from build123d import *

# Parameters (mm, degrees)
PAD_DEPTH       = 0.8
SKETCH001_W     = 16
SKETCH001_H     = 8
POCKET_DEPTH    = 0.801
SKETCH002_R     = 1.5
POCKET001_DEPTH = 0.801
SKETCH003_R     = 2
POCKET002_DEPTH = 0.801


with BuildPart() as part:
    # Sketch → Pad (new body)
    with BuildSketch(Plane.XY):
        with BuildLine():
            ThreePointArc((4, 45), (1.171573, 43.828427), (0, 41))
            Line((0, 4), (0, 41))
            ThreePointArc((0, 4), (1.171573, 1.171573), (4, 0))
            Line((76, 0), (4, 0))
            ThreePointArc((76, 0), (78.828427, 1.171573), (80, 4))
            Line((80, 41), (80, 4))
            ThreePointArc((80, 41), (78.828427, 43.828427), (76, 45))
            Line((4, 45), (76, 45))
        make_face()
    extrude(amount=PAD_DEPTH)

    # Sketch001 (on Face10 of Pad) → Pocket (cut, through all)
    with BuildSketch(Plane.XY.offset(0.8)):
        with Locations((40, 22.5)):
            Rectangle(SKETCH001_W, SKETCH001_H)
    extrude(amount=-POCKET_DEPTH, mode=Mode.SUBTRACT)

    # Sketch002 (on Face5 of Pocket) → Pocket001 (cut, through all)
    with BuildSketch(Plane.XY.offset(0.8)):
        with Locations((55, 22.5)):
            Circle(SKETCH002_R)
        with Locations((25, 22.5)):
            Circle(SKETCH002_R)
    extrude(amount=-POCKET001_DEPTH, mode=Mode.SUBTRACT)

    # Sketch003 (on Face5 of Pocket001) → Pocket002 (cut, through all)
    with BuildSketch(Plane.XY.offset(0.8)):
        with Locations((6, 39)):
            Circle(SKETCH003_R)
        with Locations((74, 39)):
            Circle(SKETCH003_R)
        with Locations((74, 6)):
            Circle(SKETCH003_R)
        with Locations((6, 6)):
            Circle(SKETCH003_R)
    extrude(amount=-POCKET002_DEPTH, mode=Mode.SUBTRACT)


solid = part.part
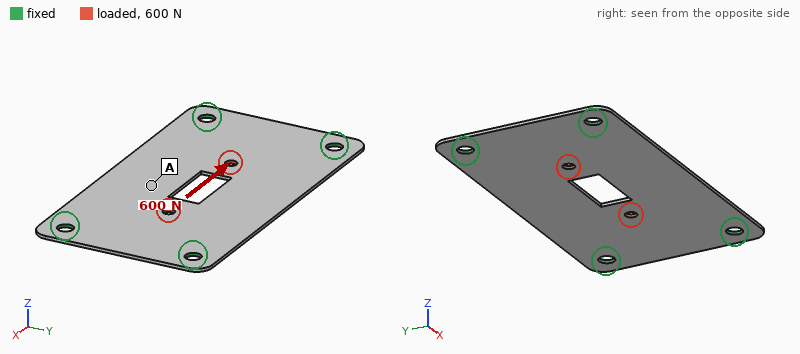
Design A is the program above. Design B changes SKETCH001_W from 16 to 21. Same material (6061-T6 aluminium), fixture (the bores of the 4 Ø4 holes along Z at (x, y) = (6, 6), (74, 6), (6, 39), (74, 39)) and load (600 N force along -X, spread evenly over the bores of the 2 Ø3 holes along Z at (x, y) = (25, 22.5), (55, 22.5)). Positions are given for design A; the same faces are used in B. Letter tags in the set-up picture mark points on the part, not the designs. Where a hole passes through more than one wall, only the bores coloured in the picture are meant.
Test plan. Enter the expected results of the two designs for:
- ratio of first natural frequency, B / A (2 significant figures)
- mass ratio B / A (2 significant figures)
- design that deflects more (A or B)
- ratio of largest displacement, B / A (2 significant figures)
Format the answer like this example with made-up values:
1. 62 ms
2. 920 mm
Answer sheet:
1. 1.0
2. 0.99
3. B
4. 1.2
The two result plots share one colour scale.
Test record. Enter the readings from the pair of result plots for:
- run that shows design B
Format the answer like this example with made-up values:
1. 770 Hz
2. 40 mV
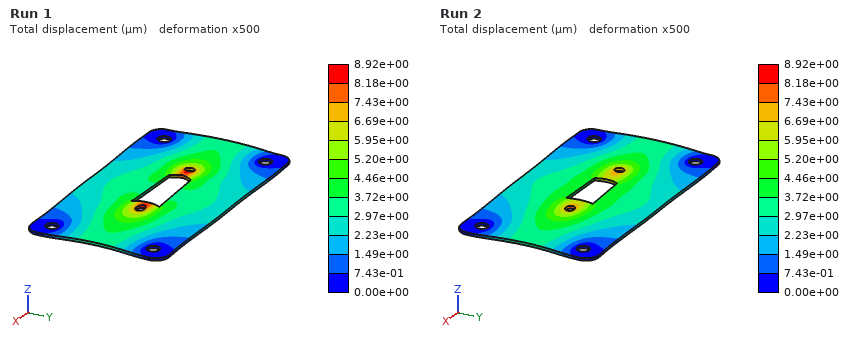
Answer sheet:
1. Run 1
